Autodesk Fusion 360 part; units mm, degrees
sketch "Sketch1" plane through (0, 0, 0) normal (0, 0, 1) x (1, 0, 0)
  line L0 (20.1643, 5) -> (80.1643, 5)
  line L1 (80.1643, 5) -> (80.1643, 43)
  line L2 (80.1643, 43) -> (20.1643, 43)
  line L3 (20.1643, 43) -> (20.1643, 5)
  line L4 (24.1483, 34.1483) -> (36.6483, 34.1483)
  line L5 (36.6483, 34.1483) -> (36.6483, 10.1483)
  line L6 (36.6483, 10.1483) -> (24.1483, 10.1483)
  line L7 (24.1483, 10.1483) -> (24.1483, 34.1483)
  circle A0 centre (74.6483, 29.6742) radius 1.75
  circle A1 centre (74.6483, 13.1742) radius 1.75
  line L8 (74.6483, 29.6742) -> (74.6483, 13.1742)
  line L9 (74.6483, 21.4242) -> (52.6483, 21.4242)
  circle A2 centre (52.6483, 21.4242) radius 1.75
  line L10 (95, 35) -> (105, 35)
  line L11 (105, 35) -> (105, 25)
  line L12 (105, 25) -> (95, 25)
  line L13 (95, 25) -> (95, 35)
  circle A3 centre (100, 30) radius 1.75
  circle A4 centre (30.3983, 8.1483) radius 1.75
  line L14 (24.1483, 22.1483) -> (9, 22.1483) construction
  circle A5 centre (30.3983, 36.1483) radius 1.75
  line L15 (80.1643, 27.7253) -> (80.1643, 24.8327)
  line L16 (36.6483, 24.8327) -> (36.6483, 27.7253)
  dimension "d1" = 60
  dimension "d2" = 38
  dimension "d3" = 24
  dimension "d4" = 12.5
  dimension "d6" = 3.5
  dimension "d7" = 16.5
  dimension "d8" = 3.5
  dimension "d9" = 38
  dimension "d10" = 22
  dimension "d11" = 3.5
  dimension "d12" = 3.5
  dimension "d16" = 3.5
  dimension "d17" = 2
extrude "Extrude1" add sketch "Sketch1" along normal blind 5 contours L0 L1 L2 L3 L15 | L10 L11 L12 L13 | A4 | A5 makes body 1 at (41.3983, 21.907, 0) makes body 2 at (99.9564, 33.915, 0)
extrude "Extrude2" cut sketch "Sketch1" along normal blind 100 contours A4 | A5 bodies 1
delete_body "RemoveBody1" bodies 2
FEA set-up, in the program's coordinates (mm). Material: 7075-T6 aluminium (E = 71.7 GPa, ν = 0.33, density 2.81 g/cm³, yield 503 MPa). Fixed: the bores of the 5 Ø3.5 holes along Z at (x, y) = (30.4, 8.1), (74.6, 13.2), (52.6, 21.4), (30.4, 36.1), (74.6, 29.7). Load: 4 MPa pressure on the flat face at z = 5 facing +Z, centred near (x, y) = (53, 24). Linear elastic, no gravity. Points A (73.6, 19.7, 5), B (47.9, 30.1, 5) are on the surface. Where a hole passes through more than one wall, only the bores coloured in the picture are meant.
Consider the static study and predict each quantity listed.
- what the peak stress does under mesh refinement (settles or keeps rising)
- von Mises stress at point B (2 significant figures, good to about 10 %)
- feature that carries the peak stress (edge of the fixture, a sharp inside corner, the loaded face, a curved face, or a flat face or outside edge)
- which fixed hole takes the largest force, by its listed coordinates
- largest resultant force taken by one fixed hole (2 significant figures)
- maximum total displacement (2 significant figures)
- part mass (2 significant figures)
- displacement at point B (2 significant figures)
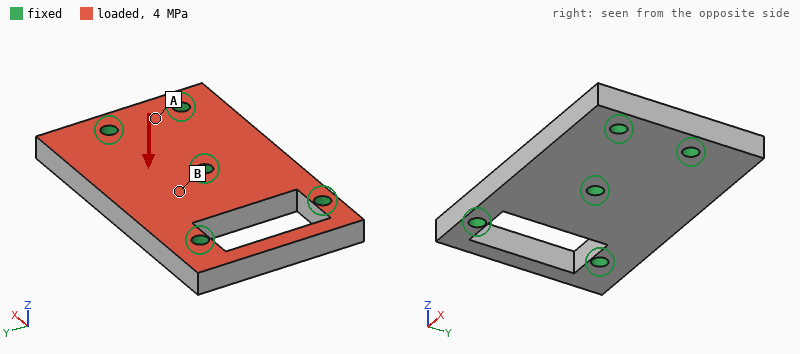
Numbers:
keeps rising
41 MPa
edge of the fixture
(52.6, 21.4)
2.7 kN
61 µm
27 g
20 µm
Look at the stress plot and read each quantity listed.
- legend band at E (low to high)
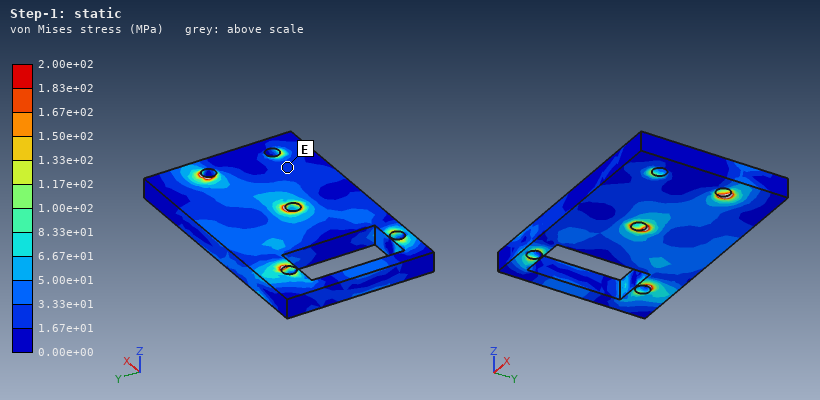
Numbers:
1.67e+01 to 3.33e+01 MPa
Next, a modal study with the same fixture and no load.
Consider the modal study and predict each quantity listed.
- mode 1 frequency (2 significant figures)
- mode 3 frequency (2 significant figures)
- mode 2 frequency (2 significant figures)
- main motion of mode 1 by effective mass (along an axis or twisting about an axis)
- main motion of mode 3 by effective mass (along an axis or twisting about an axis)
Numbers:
14 kHz
20 kHz
17 kHz
along Z
along Z
